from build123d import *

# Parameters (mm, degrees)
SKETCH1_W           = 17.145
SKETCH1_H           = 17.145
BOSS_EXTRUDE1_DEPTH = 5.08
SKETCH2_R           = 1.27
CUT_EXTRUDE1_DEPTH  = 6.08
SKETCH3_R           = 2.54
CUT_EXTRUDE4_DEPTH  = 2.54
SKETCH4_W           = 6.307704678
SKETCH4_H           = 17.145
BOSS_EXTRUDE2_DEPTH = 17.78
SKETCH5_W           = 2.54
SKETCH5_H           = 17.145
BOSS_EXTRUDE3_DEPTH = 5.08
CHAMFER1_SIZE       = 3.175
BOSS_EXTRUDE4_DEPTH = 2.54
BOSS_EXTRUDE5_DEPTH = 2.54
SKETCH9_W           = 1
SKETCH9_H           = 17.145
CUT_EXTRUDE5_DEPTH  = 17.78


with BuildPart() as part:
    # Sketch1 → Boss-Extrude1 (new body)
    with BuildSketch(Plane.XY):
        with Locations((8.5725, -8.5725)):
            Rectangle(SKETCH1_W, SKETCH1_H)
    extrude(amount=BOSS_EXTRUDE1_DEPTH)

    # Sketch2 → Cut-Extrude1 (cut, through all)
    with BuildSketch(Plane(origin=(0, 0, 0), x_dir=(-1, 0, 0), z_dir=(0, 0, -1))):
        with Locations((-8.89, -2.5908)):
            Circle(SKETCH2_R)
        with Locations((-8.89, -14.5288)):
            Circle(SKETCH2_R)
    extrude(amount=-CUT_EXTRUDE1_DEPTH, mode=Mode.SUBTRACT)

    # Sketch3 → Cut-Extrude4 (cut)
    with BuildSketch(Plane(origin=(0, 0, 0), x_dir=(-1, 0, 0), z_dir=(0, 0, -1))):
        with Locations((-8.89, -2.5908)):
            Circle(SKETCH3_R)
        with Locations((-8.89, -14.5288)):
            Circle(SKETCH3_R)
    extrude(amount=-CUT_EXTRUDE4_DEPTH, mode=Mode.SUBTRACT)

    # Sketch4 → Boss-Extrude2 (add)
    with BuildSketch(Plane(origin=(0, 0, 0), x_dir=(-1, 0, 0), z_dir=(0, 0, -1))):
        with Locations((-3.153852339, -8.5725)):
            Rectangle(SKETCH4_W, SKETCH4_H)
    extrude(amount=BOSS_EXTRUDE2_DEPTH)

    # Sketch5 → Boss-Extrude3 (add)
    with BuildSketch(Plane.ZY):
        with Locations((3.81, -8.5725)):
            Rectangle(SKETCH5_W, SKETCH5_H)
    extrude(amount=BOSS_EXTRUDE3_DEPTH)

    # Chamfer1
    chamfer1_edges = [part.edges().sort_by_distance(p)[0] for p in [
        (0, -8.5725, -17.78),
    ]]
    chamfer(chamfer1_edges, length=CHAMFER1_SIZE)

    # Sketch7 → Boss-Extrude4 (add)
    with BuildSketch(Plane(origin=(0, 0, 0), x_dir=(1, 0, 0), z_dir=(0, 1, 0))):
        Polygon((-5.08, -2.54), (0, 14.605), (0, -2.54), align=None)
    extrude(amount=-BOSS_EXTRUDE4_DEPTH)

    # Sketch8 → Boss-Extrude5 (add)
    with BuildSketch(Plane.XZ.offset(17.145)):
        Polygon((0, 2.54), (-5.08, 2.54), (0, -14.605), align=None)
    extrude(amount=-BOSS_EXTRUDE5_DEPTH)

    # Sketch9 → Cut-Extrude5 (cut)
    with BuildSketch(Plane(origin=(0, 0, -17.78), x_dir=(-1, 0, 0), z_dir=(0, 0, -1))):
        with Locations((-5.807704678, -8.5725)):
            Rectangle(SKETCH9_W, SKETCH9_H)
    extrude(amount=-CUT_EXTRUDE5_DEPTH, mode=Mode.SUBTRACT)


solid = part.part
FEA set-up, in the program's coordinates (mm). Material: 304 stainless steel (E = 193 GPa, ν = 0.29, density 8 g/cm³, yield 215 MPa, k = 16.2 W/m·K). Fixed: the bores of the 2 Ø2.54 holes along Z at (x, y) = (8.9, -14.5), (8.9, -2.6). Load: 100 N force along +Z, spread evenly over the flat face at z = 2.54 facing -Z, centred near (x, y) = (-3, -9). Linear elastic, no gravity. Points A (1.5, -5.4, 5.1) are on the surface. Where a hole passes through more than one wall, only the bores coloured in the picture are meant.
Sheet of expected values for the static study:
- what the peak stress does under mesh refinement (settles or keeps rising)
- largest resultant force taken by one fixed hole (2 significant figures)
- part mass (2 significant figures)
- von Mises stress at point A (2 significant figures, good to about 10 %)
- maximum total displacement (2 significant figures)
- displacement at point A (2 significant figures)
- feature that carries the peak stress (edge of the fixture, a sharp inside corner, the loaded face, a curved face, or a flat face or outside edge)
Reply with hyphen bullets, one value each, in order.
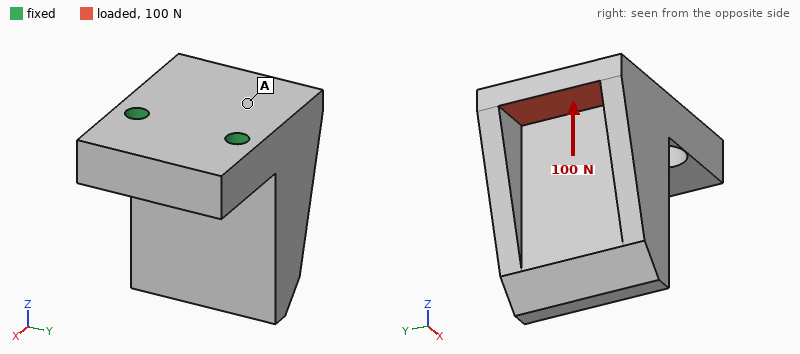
- keeps rising
- 54 N
- 27 g
- 6.7 MPa
- 8.3 µm
- 2.5 µm
- edge of the fixture
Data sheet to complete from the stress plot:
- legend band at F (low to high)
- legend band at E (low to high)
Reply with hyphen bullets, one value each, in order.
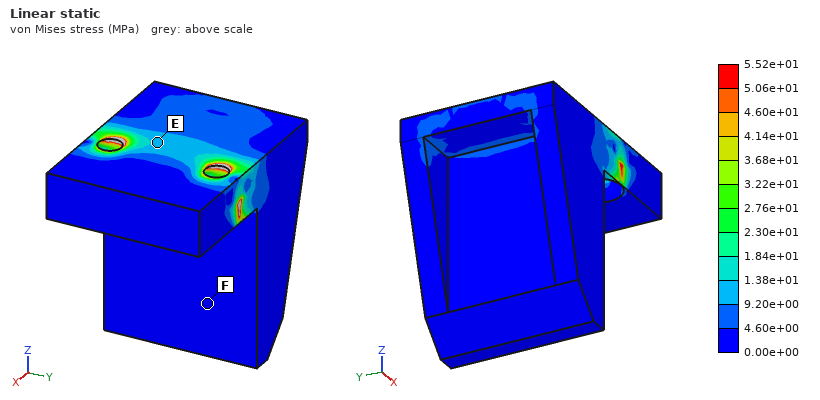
- 0.00e+00 to 4.60e+00 MPa
- 9.20e+00 to 1.38e+01 MPa
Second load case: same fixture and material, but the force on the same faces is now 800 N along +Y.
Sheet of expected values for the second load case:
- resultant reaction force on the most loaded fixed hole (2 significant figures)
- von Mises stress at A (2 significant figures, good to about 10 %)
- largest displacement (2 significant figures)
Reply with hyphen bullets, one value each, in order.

- 800 N
- 29 MPa
- 5.0 µm
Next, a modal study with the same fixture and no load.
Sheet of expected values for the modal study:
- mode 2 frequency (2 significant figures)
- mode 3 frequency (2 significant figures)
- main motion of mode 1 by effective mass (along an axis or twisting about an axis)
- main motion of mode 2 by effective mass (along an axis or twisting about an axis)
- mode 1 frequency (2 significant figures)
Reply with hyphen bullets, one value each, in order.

- 11 kHz
- 20 kHz
- along X
- along Y
- 4600 Hz
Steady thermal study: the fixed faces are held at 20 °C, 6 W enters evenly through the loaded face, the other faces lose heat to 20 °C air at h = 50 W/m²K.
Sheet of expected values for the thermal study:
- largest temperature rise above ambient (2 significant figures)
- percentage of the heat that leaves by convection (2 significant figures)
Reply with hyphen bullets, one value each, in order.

- 66 K
- 33 %
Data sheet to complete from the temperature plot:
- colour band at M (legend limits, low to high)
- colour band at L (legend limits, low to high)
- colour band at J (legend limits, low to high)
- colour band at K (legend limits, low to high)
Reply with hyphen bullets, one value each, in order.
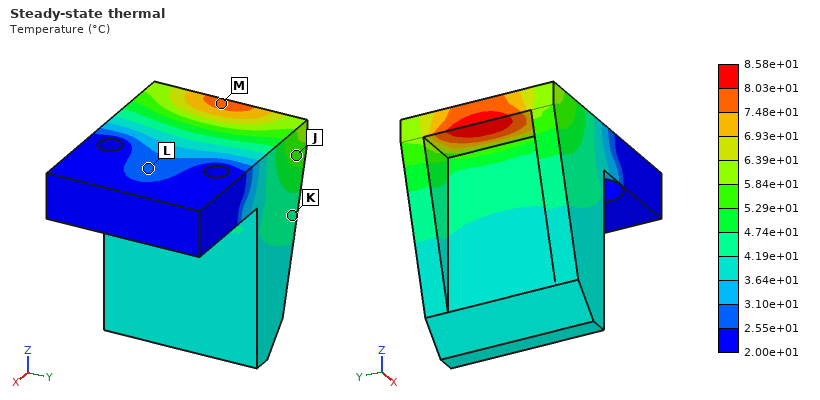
- 7.48e+01 to 8.03e+01 °C
- 2.55e+01 to 3.10e+01 °C
- 5.29e+01 to 5.84e+01 °C
- 4.19e+01 to 4.74e+01 °C
